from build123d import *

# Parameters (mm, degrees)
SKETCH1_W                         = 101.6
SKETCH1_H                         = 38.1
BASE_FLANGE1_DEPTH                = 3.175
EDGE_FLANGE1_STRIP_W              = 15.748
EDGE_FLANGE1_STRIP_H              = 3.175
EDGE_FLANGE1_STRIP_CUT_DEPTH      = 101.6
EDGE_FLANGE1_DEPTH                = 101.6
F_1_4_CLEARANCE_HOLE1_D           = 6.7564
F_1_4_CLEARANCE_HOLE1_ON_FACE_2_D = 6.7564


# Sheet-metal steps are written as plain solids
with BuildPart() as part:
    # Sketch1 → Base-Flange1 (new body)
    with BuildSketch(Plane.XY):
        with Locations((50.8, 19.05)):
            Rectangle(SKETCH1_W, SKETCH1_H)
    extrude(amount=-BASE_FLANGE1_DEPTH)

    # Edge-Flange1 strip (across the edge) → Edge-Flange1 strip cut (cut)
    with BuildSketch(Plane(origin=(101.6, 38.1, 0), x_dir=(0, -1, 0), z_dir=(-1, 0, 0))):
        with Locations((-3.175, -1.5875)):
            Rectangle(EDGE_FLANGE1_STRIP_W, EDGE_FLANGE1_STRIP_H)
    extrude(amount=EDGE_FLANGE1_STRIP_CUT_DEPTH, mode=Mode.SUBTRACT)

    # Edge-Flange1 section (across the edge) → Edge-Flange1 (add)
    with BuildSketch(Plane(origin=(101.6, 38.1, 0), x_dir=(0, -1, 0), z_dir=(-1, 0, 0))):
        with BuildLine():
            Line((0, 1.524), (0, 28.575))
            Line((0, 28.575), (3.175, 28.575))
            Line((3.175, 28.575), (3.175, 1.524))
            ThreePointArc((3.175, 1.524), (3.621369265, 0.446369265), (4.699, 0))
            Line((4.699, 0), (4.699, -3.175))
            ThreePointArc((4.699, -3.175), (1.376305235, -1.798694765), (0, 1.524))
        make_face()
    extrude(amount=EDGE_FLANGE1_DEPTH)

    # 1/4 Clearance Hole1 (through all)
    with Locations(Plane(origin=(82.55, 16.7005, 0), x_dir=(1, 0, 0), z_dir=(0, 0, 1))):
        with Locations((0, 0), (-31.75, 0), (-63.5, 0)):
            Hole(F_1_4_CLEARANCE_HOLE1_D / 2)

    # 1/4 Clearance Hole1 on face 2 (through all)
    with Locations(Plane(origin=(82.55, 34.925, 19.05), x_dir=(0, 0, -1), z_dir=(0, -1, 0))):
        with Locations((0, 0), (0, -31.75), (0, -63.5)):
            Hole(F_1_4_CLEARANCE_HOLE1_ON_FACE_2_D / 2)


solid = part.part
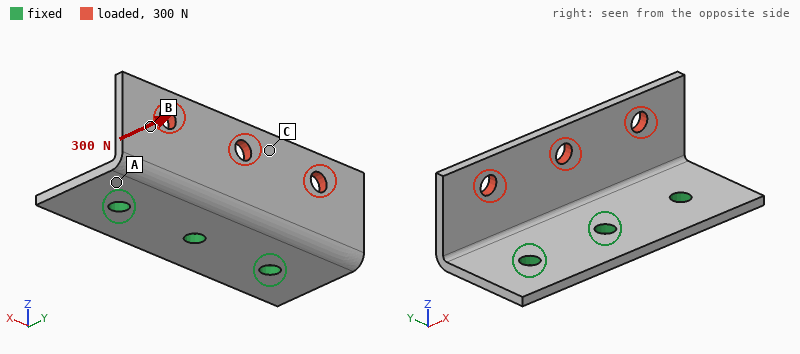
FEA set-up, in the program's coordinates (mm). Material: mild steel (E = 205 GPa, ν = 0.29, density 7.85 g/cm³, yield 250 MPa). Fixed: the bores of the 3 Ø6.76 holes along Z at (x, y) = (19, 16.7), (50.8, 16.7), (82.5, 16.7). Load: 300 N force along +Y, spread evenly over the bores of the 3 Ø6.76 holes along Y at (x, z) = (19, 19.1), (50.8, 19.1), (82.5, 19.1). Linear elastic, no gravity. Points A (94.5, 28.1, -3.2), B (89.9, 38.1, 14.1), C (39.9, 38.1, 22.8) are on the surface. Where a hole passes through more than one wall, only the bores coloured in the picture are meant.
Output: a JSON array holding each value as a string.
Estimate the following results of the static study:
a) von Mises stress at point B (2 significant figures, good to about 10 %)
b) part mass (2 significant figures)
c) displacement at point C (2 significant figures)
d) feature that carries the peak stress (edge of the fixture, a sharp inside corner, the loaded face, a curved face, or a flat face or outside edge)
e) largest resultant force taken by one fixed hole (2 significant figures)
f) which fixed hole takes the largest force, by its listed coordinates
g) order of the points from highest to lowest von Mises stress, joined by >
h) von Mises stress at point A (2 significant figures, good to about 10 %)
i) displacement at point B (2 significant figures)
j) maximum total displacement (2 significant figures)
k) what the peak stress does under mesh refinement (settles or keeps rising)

["11 MPa", "160 g", "70 µm", "edge of the fixture", "110 N", "(50.8, 16.7)", "A > B > C", "29 MPa", "45 µm", "87 µm", "keeps rising"]
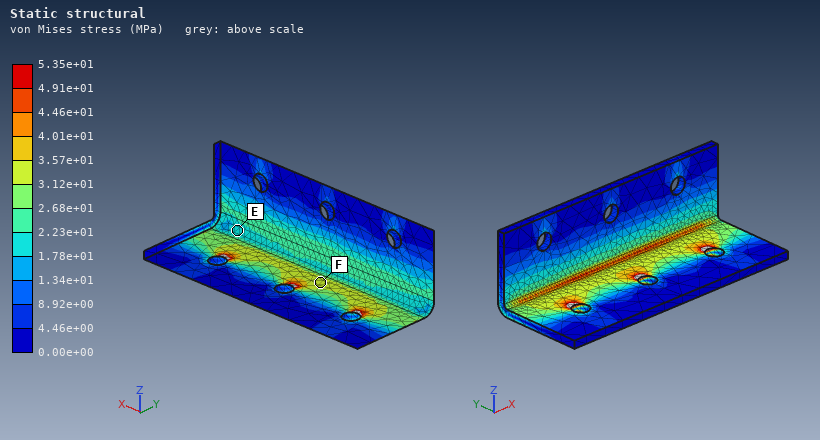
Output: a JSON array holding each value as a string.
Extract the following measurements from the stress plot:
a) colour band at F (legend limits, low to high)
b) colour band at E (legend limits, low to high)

["3.12e+01 to 3.57e+01 MPa", "1.78e+01 to 2.23e+01 MPa"]
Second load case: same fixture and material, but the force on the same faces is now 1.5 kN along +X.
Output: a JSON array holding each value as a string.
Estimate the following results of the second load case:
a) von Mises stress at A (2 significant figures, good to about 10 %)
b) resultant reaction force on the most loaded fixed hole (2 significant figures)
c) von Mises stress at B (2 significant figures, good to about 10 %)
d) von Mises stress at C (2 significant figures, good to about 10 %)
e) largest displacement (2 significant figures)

["27 MPa", "770 N", "10 MPa", "17 MPa", "94 µm"]
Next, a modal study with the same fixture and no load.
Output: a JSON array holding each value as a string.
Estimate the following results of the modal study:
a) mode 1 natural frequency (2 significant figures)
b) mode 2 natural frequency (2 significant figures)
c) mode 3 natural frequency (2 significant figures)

["1500 Hz", "2000 Hz", "4000 Hz"]
